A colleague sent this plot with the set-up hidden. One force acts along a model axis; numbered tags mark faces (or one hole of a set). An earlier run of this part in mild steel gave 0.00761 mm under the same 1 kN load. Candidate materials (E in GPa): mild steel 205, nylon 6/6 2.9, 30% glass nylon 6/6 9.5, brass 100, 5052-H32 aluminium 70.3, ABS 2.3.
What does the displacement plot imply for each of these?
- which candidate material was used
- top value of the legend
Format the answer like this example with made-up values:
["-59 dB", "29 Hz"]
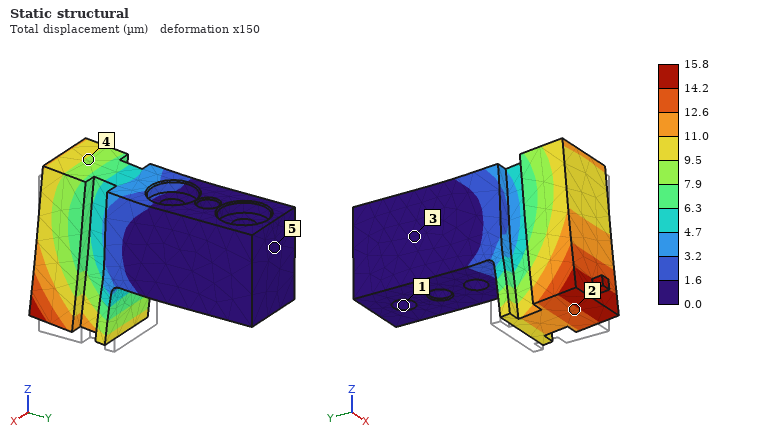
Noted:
["brass", "15.8 µm"]
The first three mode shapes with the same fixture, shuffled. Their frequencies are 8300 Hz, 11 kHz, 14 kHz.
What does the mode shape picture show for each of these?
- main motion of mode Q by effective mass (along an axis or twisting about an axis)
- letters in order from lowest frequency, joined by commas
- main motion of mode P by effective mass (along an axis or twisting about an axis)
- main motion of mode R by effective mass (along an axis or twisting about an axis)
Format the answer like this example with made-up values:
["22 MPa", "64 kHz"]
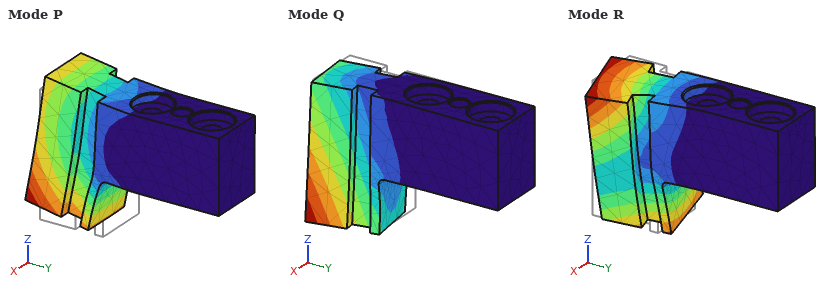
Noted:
["along X", "Q, P, R", "along Z", "twisting about Y"]
